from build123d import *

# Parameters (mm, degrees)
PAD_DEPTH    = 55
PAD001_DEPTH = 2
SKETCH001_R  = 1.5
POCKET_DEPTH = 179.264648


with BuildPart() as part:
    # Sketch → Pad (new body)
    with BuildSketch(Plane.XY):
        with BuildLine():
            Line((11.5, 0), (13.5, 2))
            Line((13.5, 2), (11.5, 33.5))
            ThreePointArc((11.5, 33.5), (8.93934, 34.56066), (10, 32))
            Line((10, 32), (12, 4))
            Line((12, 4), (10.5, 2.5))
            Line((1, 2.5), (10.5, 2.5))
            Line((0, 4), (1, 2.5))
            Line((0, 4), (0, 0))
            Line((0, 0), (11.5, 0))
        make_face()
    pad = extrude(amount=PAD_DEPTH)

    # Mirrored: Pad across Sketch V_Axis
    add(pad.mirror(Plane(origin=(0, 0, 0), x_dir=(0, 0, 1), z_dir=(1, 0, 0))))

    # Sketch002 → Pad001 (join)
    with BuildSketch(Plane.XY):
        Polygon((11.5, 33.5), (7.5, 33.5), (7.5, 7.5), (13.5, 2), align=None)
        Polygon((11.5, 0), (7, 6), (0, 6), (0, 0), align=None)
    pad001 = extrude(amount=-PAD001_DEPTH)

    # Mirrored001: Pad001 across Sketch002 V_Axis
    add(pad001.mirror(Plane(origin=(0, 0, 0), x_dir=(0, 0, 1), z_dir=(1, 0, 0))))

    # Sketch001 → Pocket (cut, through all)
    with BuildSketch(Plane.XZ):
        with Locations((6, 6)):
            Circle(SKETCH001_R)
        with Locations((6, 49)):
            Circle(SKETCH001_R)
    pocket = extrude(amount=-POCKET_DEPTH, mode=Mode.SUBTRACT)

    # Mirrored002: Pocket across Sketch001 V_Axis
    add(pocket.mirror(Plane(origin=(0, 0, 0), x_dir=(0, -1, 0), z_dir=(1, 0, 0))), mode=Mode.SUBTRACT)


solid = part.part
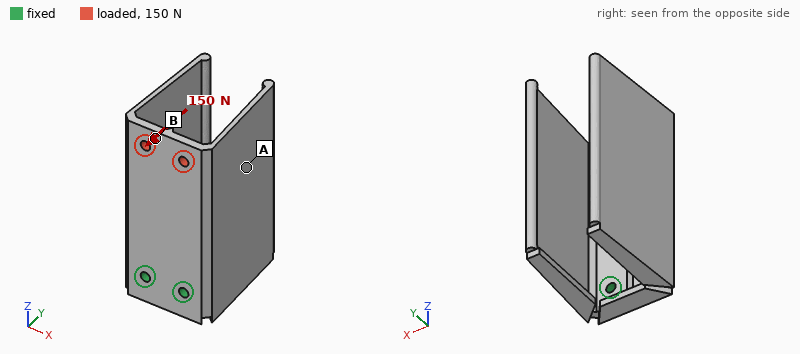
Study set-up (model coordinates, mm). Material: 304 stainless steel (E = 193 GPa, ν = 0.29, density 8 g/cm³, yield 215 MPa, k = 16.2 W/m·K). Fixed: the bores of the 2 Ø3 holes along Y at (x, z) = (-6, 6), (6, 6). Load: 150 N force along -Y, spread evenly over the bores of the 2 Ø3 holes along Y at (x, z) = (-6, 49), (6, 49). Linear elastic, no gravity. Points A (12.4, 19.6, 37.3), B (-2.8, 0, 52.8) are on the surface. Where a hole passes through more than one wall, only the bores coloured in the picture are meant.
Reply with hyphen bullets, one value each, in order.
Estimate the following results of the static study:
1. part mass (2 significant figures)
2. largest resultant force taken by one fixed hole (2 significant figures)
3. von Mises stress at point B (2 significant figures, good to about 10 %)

- 80 g
- 78 N
- 24 MPa
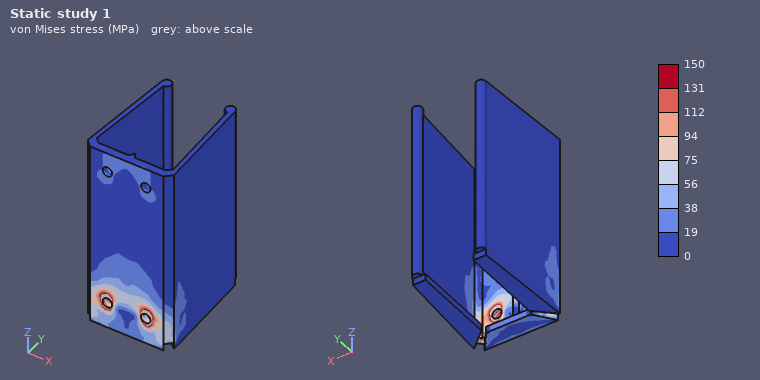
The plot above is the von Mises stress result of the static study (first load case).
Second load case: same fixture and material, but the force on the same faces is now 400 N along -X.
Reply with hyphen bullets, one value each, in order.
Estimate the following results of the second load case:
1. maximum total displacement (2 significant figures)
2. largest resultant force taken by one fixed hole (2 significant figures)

- 24 µm
- 1.2 kN
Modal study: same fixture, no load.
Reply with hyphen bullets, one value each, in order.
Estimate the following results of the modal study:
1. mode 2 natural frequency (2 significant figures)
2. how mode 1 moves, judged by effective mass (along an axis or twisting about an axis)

- 950 Hz
- along X
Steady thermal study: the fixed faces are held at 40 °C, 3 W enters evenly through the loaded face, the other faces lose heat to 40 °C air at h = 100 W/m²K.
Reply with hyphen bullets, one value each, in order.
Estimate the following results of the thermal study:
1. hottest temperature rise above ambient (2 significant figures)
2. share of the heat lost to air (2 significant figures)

- 25 K
- 97 %
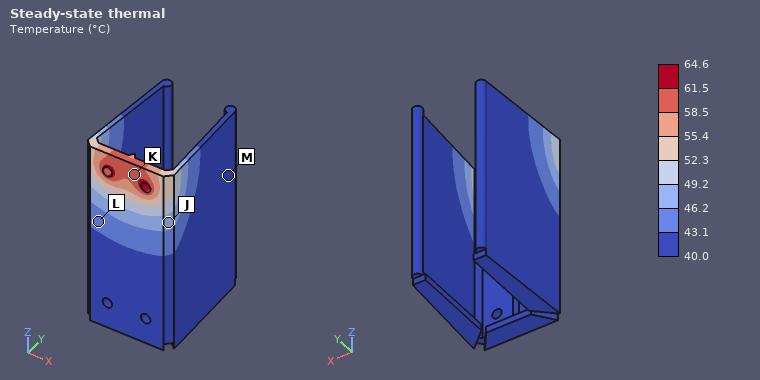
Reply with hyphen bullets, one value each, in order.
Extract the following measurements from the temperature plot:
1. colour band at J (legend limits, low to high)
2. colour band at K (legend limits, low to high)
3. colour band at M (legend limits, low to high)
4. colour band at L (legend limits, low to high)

- 46.2 to 49.2 °C
- 58.5 to 61.5 °C
- 40.0 to 43.1 °C
- 43.1 to 46.2 °C
